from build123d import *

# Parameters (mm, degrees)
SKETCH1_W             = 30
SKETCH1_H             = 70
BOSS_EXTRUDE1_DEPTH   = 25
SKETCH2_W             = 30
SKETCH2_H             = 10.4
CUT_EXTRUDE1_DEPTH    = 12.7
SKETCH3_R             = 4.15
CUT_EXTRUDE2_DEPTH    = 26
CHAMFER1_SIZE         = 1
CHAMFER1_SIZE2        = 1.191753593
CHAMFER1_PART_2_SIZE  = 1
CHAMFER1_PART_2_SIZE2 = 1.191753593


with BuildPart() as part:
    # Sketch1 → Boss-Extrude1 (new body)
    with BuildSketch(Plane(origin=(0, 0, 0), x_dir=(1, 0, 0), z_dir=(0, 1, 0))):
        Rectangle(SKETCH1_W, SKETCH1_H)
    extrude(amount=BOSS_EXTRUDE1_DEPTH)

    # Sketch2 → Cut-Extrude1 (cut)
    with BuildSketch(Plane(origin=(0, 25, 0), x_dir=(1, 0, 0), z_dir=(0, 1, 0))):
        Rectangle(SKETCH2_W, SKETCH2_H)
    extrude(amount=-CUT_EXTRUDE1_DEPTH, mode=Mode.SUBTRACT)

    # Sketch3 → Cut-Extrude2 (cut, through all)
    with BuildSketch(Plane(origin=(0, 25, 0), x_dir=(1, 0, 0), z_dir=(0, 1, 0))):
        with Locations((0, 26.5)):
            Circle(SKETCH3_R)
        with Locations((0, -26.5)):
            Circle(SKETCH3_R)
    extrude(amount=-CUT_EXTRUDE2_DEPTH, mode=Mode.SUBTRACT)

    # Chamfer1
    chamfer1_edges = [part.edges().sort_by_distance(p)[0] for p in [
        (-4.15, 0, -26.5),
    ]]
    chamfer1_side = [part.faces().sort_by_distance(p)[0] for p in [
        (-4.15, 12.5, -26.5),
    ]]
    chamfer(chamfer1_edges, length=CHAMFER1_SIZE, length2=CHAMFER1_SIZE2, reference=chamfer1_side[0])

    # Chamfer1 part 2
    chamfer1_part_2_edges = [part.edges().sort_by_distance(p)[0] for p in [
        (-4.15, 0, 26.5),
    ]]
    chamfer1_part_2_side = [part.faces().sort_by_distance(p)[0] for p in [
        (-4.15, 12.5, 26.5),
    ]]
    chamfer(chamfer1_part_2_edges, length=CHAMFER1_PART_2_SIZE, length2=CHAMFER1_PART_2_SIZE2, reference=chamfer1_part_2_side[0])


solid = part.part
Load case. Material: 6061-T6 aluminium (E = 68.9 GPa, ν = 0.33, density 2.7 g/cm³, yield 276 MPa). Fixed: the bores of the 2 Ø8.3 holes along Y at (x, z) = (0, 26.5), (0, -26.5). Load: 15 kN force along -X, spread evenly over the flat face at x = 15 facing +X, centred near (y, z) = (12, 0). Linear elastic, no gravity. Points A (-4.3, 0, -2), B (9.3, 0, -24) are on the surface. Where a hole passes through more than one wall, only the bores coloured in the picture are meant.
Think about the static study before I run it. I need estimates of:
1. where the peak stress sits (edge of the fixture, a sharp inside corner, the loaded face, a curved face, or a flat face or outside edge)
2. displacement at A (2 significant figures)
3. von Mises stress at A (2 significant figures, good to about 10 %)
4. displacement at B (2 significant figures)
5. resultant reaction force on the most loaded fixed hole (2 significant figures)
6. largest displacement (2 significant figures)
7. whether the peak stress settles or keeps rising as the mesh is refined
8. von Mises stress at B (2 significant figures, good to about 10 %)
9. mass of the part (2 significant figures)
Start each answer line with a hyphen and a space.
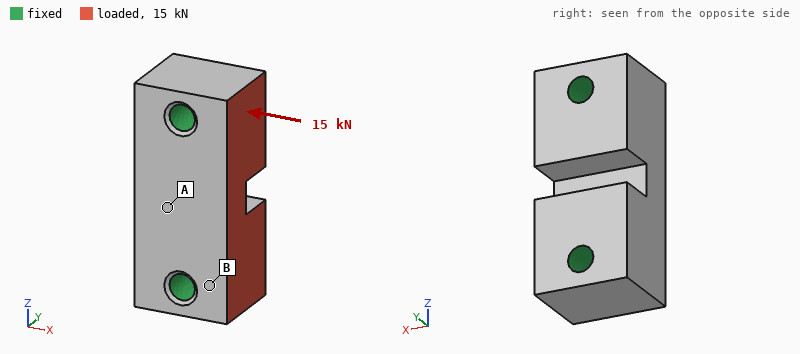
- edge of the fixture
- 7.6 µm
- 5.0 MPa
- 2.2 µm
- 7.5 kN
- 9.5 µm
- keeps rising
- 13 MPa
- 120 g
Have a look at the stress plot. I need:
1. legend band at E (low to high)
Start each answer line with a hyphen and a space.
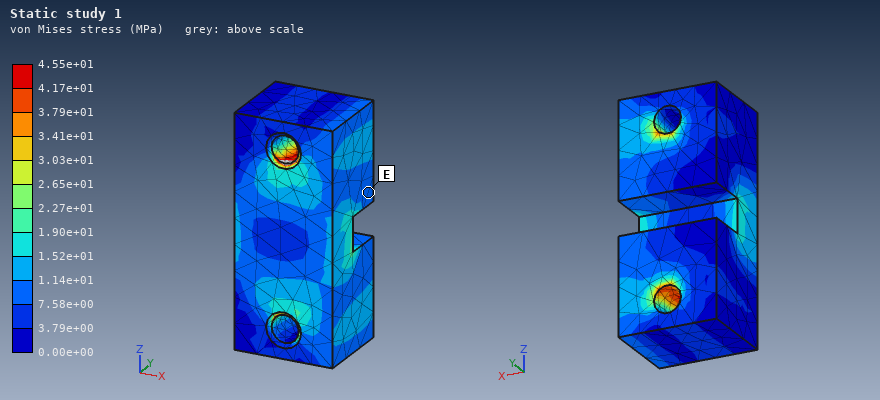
- 7.58e+00 to 1.14e+01 MPa
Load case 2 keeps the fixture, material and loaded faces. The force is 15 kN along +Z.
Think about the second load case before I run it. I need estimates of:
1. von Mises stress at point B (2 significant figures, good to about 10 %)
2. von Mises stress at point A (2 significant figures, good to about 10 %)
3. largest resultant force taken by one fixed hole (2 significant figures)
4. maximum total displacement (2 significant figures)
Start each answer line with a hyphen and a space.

- 21 MPa
- 6.8 MPa
- 8.1 kN
- 13 µm
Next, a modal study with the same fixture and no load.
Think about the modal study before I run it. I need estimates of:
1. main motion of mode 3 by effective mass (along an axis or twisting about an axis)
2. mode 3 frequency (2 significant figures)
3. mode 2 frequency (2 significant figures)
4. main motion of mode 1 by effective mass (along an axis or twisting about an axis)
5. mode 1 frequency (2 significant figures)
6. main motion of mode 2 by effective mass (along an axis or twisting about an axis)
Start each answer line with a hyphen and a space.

- twisting about Z
- 28 kHz
- 23 kHz
- along X
- 21 kHz
- along Y
